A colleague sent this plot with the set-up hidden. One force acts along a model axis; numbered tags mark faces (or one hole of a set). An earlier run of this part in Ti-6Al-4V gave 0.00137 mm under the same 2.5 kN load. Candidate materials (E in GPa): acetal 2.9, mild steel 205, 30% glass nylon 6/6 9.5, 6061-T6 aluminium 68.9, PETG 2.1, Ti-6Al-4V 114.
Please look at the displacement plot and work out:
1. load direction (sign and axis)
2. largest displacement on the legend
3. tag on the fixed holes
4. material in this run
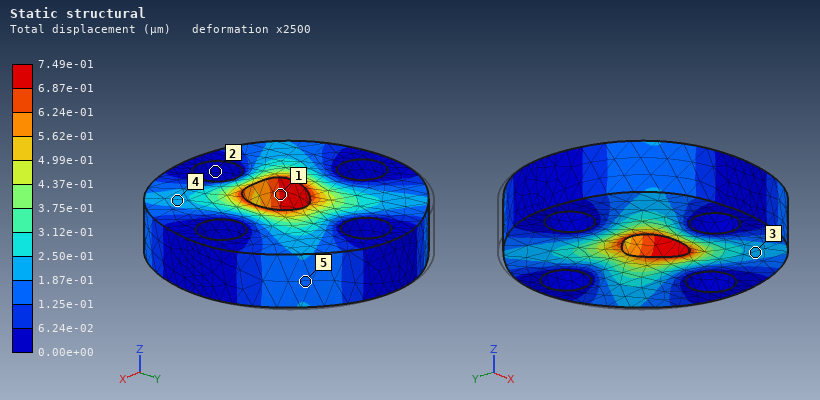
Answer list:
-Y
7.49e-01 µm
2
mild steel
